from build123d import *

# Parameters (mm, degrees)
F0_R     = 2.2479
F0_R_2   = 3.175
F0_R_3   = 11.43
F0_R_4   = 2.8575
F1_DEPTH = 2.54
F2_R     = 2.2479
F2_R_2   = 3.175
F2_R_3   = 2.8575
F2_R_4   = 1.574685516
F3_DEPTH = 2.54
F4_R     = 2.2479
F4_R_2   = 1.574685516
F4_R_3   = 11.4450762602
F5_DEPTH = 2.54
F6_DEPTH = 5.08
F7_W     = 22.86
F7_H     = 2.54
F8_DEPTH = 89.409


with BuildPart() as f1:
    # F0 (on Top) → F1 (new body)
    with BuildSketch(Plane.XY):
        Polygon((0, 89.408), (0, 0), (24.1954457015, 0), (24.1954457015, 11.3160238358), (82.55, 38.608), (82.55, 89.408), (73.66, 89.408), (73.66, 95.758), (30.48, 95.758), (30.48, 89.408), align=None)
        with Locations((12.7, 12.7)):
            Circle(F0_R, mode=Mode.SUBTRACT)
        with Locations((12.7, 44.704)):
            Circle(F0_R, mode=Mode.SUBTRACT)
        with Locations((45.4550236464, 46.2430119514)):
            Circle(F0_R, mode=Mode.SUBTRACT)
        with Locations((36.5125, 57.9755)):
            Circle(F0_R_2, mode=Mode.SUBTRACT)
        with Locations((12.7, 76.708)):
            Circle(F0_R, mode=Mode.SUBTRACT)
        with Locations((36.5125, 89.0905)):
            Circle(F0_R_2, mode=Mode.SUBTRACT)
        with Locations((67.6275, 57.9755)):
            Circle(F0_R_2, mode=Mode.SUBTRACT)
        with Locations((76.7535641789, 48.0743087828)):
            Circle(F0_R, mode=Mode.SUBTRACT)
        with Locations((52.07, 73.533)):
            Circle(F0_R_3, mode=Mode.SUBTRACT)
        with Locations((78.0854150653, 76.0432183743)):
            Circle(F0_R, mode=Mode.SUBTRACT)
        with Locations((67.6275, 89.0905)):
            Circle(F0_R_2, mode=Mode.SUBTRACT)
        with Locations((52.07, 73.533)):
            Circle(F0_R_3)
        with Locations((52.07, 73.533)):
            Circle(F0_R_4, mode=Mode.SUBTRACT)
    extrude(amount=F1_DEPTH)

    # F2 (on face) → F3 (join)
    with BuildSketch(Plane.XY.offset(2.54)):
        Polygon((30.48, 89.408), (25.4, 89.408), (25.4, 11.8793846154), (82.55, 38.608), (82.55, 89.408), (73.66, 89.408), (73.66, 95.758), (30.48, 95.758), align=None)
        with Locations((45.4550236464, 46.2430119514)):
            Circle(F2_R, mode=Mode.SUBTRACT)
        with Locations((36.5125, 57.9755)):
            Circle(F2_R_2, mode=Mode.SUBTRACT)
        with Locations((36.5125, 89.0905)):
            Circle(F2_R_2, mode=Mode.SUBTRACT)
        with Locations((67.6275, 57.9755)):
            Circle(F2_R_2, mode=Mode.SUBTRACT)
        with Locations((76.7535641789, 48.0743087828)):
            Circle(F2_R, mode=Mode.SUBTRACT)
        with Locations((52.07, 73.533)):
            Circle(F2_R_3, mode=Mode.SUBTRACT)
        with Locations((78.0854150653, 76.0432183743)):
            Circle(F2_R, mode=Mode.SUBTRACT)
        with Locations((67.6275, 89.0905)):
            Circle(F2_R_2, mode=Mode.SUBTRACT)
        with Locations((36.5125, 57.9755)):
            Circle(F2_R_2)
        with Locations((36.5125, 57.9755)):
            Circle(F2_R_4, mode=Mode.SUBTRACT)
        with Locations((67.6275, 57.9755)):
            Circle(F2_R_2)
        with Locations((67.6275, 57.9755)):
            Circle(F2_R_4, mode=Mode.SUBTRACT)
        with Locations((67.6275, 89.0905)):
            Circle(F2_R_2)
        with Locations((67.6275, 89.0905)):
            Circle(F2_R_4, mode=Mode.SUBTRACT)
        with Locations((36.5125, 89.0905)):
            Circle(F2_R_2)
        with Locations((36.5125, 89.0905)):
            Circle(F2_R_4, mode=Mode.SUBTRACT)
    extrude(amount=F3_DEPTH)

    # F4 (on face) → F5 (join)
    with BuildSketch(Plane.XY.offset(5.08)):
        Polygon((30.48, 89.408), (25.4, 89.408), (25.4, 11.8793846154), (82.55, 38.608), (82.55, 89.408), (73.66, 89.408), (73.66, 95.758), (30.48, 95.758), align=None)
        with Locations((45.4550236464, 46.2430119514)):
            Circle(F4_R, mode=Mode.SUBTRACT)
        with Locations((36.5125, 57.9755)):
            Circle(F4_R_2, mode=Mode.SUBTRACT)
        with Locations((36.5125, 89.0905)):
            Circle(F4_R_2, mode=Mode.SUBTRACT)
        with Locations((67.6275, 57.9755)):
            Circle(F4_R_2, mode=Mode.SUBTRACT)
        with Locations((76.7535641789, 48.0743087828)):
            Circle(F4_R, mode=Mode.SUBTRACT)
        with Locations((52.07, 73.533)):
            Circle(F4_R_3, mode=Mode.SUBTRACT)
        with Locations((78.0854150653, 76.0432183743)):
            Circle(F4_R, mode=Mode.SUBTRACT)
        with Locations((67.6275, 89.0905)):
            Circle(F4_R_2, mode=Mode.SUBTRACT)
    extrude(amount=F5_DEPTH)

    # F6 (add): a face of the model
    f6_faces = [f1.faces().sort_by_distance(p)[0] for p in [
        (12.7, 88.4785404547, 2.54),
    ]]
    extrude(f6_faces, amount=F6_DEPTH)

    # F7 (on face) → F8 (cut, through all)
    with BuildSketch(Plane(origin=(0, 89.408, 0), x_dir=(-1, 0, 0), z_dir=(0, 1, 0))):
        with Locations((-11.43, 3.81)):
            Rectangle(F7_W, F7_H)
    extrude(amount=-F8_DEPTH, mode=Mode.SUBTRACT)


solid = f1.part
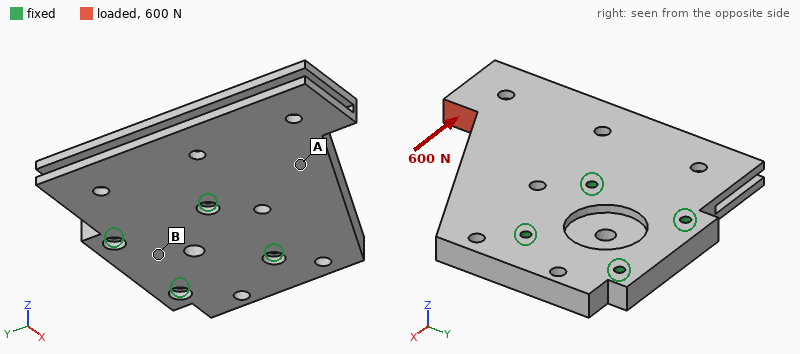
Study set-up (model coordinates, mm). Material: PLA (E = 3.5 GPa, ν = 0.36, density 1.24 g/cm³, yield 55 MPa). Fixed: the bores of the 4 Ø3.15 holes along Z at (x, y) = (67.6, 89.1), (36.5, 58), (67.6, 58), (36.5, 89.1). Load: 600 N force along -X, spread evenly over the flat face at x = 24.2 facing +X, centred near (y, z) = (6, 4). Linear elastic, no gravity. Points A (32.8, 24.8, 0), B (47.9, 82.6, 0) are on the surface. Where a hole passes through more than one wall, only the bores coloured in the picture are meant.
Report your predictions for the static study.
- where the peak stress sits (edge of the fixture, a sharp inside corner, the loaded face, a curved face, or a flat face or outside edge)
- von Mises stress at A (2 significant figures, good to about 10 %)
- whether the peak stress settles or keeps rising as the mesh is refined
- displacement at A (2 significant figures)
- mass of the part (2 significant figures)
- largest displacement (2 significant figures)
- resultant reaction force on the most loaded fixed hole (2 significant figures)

edge of the fixture
5.2 MPa
keeps rising
0.12 mm
49 g
0.39 mm
680 N
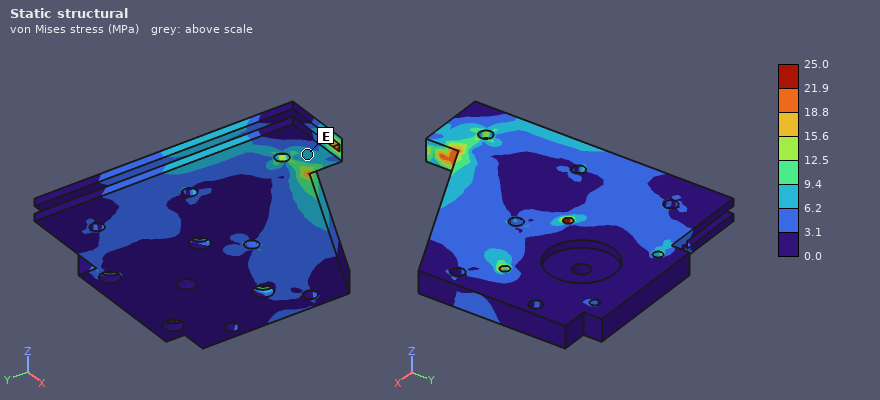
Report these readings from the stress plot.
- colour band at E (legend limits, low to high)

6.2 to 9.4 MPa
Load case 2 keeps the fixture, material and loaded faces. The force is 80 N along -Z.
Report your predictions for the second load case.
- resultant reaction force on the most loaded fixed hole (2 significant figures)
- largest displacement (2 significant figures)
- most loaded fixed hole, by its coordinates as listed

200 N
1.4 mm
(36.5, 58)
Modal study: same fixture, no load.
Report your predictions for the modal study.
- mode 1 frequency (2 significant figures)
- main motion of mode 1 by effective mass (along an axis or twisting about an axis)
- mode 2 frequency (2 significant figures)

570 Hz
along Z
1000 Hz
